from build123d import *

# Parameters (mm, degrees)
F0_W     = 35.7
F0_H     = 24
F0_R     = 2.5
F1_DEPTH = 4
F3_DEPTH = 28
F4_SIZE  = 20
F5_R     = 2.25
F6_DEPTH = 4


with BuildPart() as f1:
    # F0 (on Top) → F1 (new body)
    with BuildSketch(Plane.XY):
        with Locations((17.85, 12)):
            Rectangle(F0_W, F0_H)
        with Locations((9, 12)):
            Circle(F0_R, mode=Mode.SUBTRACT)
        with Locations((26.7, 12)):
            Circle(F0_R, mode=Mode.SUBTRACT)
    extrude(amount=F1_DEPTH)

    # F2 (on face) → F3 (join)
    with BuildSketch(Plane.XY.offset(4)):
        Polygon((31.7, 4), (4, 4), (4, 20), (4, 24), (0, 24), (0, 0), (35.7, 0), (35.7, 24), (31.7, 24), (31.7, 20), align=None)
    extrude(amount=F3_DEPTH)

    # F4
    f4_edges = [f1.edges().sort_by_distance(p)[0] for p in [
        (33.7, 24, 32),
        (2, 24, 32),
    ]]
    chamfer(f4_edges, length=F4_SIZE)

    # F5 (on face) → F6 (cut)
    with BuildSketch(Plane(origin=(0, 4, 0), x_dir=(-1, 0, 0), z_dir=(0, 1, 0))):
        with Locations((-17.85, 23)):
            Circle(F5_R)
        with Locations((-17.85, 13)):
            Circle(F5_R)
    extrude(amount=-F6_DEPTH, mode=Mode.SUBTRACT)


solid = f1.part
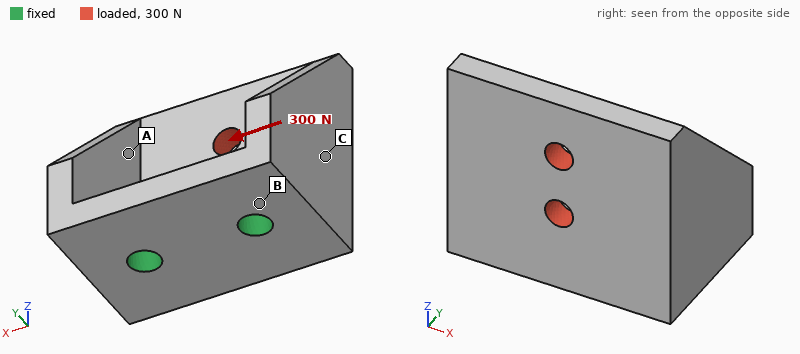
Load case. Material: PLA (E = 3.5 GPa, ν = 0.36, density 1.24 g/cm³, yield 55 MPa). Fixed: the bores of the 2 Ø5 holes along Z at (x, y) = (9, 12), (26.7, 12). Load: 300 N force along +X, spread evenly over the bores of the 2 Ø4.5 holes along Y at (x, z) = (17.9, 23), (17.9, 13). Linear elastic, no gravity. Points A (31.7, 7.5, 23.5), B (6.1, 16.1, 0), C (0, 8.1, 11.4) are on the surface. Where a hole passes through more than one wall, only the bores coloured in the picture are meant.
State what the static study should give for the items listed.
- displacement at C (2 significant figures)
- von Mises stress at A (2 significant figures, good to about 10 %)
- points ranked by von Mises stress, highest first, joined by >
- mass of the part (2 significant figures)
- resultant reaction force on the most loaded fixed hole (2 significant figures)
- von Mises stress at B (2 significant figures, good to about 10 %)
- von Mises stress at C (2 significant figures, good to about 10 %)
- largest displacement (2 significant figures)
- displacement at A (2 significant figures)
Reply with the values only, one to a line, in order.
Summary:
0.13 mm
4.3 MPa
B > A > C
12 g
270 N
7.8 MPa
2.6 MPa
0.31 mm
0.23 mm
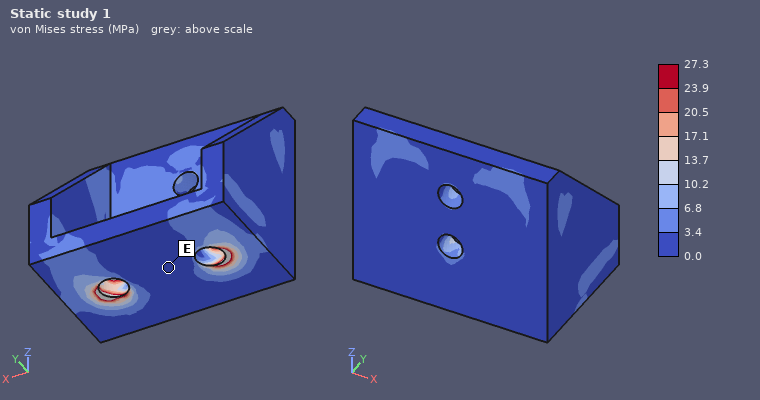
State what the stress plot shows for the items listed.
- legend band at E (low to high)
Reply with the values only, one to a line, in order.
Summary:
0.0 to 3.4 MPa
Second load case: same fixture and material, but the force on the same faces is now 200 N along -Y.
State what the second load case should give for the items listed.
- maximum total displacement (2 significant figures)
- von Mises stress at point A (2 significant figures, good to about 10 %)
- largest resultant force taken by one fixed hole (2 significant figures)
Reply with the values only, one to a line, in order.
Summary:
0.50 mm
5.3 MPa
110 N
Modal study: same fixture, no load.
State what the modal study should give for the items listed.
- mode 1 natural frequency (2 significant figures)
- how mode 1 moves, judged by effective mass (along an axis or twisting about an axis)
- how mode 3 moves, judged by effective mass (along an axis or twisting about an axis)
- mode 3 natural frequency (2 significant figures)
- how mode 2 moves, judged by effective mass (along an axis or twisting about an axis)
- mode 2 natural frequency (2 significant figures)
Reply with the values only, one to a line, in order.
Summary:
1600 Hz
along Y
along X
3800 Hz
along X
1900 Hz
